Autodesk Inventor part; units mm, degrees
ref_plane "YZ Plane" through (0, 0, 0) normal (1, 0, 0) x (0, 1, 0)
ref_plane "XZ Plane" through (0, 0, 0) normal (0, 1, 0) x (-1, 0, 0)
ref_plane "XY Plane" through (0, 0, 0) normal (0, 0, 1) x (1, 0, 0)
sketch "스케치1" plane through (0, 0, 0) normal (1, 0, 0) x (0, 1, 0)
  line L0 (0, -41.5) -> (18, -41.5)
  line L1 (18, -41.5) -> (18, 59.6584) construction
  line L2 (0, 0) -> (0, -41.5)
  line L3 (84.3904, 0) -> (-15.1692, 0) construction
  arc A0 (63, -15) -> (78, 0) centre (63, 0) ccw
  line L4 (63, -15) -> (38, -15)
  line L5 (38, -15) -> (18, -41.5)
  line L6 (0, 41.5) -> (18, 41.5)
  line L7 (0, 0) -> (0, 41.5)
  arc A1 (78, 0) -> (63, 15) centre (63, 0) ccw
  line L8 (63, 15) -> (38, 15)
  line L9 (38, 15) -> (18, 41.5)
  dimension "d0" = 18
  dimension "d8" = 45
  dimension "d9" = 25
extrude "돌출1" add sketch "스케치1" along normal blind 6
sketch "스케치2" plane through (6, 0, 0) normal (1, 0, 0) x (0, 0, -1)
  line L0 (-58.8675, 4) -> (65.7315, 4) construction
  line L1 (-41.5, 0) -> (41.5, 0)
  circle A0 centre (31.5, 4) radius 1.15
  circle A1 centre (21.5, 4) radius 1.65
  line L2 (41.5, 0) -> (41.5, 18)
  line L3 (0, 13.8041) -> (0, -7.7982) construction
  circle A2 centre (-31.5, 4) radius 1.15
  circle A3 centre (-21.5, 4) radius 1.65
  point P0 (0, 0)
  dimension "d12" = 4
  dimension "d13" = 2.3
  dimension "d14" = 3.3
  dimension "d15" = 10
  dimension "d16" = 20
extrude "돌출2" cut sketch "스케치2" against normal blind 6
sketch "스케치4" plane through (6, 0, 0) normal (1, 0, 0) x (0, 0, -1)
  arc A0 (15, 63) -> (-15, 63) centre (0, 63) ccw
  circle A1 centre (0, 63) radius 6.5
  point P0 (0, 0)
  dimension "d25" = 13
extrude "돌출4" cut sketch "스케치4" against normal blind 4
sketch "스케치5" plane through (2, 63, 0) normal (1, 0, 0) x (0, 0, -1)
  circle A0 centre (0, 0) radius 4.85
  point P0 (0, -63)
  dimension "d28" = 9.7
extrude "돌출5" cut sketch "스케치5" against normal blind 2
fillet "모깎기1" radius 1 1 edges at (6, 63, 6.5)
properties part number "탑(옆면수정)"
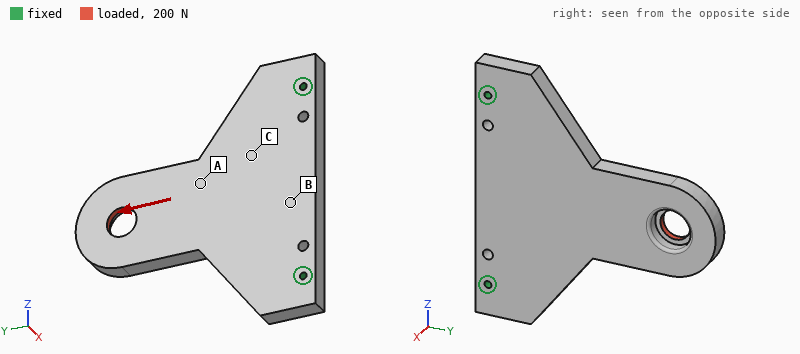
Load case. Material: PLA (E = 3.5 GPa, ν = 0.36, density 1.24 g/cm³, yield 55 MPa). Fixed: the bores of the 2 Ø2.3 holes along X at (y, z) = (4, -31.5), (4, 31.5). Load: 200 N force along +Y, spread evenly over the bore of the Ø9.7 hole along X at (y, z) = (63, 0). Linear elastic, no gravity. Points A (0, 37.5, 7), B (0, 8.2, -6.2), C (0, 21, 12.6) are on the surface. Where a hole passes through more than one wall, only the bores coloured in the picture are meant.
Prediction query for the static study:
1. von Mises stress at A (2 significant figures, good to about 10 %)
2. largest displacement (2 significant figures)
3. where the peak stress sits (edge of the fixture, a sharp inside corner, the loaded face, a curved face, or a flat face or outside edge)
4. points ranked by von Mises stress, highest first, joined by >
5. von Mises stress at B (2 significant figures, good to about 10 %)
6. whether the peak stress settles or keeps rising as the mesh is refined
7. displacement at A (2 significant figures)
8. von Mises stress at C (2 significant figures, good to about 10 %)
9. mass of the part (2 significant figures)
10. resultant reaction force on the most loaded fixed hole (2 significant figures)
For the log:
2.7 MPa
0.51 mm
edge of the fixture
A > C > B
0.65 MPa
keeps rising
0.12 mm
1.8 MPa
27 g
110 N
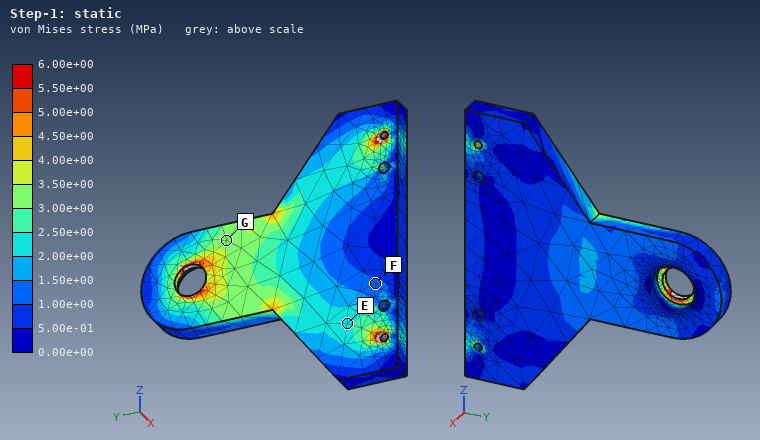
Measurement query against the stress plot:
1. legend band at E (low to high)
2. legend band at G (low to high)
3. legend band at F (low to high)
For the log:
2.00e+00 to 2.50e+00 MPa
3.00e+00 to 3.50e+00 MPa
1.00e+00 to 1.50e+00 MPa
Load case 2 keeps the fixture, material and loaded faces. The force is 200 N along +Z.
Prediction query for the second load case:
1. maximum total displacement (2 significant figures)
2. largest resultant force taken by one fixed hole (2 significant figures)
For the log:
0.20 mm
210 N
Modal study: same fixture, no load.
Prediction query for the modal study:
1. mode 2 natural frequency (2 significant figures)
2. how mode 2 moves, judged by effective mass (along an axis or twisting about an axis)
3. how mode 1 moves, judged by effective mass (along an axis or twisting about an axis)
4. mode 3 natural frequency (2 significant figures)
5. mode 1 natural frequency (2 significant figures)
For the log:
1500 Hz
along X
along X
1800 Hz
340 Hz
